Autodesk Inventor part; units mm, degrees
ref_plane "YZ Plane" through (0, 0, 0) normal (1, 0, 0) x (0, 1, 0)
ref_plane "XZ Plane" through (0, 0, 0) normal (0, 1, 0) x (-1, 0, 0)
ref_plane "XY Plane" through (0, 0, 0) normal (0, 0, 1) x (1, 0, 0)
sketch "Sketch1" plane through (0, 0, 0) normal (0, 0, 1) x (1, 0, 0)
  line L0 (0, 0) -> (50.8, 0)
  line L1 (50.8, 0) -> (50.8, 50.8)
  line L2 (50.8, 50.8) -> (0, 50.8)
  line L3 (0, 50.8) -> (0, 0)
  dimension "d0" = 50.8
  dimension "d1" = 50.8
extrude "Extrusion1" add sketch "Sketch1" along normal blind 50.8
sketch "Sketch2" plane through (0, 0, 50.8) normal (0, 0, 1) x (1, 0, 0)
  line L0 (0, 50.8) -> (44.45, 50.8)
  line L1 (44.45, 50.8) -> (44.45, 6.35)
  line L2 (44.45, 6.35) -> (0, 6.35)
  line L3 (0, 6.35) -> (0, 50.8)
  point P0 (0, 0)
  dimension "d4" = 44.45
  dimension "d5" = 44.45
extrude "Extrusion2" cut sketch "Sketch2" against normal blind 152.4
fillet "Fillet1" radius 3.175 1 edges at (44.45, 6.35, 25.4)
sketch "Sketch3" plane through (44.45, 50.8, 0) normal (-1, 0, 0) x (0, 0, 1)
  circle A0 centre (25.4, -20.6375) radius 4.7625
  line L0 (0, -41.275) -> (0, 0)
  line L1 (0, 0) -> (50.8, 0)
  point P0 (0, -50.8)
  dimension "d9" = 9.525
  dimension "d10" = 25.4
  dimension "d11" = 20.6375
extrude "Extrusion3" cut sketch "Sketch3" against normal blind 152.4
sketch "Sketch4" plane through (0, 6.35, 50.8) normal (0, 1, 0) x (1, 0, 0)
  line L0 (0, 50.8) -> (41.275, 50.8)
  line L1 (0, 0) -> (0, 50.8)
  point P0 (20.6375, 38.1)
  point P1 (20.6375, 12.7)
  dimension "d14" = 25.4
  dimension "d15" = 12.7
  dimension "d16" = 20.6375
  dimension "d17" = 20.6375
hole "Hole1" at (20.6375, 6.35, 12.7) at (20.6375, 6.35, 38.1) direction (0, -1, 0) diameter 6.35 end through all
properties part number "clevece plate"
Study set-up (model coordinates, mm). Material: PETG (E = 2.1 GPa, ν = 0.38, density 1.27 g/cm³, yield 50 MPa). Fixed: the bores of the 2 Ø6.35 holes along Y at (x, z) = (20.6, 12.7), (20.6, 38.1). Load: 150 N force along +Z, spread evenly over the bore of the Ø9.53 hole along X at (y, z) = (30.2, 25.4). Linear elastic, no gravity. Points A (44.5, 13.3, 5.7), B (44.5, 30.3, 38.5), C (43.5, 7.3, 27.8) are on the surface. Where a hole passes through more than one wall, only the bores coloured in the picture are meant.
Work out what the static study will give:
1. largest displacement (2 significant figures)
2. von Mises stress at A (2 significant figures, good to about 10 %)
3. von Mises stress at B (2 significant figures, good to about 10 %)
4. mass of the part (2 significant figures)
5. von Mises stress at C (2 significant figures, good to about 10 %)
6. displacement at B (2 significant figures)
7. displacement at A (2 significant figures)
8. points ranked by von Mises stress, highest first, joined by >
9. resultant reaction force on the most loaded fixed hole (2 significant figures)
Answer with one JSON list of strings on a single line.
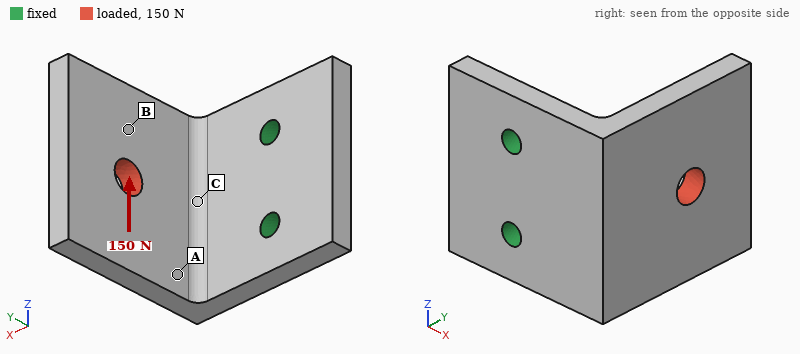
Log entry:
["0.82 mm", "4.0 MPa", "1.4 MPa", "38 g", "7.6 MPa", "0.47 mm", "0.32 mm", "C > A > B", "200 N"]
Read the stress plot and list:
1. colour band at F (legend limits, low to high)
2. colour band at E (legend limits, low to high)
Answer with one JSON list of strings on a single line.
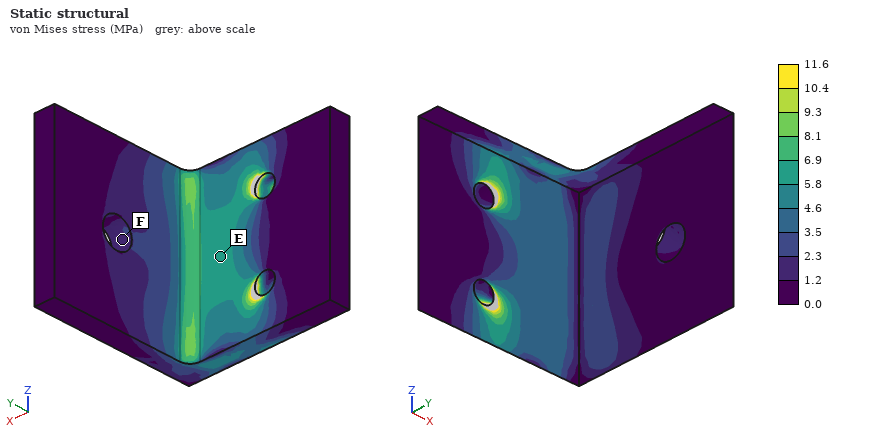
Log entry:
["1.2 to 2.3 MPa", "5.8 to 6.9 MPa"]
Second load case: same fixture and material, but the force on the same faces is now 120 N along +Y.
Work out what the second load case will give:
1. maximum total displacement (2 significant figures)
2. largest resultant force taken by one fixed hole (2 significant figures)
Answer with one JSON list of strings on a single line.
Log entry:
["0.89 mm", "60 N"]
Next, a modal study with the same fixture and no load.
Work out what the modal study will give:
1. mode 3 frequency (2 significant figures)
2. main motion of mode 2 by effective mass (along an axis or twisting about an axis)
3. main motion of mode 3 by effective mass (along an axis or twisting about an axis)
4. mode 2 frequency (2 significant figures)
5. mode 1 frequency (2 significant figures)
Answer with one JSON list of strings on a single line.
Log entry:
["1000 Hz", "along Z", "along Y", "590 Hz", "330 Hz"]
